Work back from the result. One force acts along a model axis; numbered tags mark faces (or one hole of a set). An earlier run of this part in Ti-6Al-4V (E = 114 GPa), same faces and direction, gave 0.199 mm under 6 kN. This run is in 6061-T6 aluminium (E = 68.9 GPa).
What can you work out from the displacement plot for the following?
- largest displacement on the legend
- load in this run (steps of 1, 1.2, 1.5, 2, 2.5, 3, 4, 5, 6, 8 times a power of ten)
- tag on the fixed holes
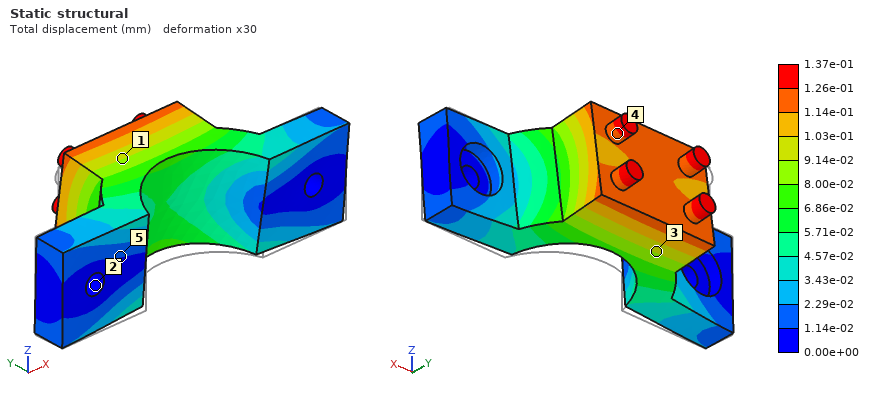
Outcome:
1.37e-01 mm
2.5 kN
2
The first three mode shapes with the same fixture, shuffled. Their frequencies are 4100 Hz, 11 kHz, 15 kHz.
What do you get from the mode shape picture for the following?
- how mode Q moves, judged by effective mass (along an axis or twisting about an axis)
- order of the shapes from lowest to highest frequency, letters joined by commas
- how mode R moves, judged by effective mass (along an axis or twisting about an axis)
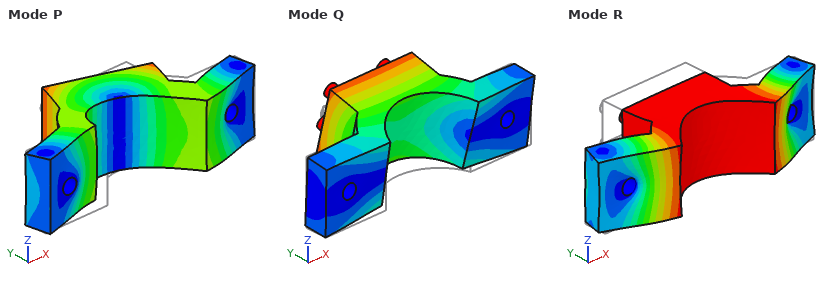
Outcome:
along Z
Q, R, P
along Y
